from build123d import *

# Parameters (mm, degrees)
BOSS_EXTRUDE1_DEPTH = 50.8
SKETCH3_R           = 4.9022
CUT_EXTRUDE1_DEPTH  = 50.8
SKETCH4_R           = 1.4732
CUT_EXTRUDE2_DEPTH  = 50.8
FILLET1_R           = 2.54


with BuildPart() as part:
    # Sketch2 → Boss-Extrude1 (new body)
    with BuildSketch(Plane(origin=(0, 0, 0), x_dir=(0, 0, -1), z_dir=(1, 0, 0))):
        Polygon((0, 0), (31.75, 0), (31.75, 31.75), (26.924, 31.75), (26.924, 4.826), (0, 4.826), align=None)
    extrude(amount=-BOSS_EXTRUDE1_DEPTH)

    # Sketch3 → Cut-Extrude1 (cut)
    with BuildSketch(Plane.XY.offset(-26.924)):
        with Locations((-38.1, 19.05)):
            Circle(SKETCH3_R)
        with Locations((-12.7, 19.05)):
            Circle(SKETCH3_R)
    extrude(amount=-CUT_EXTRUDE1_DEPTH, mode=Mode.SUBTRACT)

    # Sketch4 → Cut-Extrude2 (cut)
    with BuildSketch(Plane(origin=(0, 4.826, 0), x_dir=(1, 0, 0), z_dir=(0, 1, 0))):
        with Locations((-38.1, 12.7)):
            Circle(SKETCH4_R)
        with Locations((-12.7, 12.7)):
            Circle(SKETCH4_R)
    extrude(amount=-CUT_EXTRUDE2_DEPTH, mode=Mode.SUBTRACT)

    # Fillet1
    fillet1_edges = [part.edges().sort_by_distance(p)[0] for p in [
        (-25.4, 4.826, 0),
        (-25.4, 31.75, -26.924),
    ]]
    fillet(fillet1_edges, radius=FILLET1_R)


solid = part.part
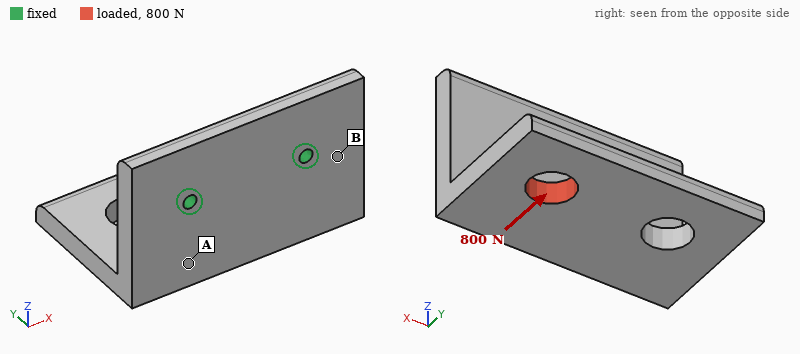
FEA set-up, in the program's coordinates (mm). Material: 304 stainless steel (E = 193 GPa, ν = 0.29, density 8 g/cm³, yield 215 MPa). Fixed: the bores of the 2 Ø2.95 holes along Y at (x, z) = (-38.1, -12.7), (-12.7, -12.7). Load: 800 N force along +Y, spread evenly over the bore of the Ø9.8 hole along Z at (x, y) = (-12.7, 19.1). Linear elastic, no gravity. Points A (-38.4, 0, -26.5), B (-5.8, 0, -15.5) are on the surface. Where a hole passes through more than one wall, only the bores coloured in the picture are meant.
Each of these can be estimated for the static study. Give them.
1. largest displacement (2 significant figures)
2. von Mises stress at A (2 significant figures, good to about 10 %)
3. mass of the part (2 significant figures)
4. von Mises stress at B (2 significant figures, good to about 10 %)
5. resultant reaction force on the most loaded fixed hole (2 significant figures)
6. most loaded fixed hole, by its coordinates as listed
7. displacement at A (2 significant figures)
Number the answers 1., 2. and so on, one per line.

1. 66 µm
2. 22 MPa
3. 110 g
4. 53 MPa
5. 730 N
6. (-12.7, -12.7)
7. 11 µm
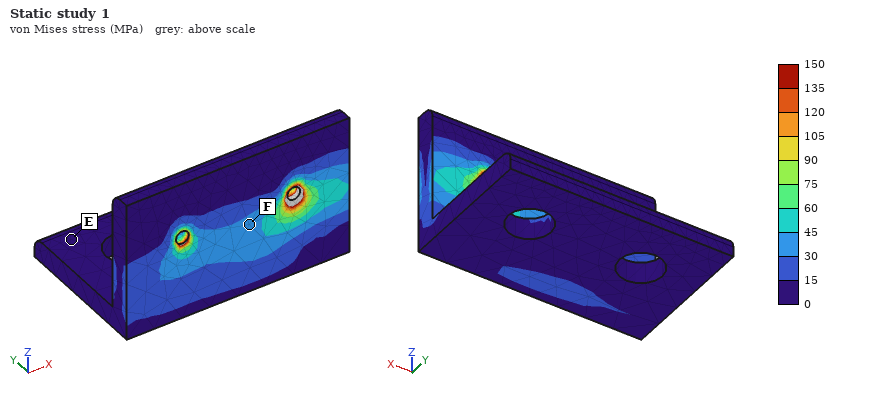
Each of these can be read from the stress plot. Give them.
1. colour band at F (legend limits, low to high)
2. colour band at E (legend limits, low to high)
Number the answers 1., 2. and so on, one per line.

1. 30 to 45 MPa
2. 0 to 15 MPa
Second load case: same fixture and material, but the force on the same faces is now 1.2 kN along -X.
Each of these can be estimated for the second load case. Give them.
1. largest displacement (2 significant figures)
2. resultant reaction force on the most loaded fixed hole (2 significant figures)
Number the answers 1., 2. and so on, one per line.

1. 42 µm
2. 1.1 kN
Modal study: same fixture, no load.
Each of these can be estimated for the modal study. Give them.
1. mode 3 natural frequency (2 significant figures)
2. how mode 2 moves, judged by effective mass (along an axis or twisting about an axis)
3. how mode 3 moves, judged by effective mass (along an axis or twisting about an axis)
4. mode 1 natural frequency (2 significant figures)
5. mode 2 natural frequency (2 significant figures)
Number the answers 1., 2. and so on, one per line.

1. 6500 Hz
2. along X
3. along Y
4. 2300 Hz
5. 4000 Hz
